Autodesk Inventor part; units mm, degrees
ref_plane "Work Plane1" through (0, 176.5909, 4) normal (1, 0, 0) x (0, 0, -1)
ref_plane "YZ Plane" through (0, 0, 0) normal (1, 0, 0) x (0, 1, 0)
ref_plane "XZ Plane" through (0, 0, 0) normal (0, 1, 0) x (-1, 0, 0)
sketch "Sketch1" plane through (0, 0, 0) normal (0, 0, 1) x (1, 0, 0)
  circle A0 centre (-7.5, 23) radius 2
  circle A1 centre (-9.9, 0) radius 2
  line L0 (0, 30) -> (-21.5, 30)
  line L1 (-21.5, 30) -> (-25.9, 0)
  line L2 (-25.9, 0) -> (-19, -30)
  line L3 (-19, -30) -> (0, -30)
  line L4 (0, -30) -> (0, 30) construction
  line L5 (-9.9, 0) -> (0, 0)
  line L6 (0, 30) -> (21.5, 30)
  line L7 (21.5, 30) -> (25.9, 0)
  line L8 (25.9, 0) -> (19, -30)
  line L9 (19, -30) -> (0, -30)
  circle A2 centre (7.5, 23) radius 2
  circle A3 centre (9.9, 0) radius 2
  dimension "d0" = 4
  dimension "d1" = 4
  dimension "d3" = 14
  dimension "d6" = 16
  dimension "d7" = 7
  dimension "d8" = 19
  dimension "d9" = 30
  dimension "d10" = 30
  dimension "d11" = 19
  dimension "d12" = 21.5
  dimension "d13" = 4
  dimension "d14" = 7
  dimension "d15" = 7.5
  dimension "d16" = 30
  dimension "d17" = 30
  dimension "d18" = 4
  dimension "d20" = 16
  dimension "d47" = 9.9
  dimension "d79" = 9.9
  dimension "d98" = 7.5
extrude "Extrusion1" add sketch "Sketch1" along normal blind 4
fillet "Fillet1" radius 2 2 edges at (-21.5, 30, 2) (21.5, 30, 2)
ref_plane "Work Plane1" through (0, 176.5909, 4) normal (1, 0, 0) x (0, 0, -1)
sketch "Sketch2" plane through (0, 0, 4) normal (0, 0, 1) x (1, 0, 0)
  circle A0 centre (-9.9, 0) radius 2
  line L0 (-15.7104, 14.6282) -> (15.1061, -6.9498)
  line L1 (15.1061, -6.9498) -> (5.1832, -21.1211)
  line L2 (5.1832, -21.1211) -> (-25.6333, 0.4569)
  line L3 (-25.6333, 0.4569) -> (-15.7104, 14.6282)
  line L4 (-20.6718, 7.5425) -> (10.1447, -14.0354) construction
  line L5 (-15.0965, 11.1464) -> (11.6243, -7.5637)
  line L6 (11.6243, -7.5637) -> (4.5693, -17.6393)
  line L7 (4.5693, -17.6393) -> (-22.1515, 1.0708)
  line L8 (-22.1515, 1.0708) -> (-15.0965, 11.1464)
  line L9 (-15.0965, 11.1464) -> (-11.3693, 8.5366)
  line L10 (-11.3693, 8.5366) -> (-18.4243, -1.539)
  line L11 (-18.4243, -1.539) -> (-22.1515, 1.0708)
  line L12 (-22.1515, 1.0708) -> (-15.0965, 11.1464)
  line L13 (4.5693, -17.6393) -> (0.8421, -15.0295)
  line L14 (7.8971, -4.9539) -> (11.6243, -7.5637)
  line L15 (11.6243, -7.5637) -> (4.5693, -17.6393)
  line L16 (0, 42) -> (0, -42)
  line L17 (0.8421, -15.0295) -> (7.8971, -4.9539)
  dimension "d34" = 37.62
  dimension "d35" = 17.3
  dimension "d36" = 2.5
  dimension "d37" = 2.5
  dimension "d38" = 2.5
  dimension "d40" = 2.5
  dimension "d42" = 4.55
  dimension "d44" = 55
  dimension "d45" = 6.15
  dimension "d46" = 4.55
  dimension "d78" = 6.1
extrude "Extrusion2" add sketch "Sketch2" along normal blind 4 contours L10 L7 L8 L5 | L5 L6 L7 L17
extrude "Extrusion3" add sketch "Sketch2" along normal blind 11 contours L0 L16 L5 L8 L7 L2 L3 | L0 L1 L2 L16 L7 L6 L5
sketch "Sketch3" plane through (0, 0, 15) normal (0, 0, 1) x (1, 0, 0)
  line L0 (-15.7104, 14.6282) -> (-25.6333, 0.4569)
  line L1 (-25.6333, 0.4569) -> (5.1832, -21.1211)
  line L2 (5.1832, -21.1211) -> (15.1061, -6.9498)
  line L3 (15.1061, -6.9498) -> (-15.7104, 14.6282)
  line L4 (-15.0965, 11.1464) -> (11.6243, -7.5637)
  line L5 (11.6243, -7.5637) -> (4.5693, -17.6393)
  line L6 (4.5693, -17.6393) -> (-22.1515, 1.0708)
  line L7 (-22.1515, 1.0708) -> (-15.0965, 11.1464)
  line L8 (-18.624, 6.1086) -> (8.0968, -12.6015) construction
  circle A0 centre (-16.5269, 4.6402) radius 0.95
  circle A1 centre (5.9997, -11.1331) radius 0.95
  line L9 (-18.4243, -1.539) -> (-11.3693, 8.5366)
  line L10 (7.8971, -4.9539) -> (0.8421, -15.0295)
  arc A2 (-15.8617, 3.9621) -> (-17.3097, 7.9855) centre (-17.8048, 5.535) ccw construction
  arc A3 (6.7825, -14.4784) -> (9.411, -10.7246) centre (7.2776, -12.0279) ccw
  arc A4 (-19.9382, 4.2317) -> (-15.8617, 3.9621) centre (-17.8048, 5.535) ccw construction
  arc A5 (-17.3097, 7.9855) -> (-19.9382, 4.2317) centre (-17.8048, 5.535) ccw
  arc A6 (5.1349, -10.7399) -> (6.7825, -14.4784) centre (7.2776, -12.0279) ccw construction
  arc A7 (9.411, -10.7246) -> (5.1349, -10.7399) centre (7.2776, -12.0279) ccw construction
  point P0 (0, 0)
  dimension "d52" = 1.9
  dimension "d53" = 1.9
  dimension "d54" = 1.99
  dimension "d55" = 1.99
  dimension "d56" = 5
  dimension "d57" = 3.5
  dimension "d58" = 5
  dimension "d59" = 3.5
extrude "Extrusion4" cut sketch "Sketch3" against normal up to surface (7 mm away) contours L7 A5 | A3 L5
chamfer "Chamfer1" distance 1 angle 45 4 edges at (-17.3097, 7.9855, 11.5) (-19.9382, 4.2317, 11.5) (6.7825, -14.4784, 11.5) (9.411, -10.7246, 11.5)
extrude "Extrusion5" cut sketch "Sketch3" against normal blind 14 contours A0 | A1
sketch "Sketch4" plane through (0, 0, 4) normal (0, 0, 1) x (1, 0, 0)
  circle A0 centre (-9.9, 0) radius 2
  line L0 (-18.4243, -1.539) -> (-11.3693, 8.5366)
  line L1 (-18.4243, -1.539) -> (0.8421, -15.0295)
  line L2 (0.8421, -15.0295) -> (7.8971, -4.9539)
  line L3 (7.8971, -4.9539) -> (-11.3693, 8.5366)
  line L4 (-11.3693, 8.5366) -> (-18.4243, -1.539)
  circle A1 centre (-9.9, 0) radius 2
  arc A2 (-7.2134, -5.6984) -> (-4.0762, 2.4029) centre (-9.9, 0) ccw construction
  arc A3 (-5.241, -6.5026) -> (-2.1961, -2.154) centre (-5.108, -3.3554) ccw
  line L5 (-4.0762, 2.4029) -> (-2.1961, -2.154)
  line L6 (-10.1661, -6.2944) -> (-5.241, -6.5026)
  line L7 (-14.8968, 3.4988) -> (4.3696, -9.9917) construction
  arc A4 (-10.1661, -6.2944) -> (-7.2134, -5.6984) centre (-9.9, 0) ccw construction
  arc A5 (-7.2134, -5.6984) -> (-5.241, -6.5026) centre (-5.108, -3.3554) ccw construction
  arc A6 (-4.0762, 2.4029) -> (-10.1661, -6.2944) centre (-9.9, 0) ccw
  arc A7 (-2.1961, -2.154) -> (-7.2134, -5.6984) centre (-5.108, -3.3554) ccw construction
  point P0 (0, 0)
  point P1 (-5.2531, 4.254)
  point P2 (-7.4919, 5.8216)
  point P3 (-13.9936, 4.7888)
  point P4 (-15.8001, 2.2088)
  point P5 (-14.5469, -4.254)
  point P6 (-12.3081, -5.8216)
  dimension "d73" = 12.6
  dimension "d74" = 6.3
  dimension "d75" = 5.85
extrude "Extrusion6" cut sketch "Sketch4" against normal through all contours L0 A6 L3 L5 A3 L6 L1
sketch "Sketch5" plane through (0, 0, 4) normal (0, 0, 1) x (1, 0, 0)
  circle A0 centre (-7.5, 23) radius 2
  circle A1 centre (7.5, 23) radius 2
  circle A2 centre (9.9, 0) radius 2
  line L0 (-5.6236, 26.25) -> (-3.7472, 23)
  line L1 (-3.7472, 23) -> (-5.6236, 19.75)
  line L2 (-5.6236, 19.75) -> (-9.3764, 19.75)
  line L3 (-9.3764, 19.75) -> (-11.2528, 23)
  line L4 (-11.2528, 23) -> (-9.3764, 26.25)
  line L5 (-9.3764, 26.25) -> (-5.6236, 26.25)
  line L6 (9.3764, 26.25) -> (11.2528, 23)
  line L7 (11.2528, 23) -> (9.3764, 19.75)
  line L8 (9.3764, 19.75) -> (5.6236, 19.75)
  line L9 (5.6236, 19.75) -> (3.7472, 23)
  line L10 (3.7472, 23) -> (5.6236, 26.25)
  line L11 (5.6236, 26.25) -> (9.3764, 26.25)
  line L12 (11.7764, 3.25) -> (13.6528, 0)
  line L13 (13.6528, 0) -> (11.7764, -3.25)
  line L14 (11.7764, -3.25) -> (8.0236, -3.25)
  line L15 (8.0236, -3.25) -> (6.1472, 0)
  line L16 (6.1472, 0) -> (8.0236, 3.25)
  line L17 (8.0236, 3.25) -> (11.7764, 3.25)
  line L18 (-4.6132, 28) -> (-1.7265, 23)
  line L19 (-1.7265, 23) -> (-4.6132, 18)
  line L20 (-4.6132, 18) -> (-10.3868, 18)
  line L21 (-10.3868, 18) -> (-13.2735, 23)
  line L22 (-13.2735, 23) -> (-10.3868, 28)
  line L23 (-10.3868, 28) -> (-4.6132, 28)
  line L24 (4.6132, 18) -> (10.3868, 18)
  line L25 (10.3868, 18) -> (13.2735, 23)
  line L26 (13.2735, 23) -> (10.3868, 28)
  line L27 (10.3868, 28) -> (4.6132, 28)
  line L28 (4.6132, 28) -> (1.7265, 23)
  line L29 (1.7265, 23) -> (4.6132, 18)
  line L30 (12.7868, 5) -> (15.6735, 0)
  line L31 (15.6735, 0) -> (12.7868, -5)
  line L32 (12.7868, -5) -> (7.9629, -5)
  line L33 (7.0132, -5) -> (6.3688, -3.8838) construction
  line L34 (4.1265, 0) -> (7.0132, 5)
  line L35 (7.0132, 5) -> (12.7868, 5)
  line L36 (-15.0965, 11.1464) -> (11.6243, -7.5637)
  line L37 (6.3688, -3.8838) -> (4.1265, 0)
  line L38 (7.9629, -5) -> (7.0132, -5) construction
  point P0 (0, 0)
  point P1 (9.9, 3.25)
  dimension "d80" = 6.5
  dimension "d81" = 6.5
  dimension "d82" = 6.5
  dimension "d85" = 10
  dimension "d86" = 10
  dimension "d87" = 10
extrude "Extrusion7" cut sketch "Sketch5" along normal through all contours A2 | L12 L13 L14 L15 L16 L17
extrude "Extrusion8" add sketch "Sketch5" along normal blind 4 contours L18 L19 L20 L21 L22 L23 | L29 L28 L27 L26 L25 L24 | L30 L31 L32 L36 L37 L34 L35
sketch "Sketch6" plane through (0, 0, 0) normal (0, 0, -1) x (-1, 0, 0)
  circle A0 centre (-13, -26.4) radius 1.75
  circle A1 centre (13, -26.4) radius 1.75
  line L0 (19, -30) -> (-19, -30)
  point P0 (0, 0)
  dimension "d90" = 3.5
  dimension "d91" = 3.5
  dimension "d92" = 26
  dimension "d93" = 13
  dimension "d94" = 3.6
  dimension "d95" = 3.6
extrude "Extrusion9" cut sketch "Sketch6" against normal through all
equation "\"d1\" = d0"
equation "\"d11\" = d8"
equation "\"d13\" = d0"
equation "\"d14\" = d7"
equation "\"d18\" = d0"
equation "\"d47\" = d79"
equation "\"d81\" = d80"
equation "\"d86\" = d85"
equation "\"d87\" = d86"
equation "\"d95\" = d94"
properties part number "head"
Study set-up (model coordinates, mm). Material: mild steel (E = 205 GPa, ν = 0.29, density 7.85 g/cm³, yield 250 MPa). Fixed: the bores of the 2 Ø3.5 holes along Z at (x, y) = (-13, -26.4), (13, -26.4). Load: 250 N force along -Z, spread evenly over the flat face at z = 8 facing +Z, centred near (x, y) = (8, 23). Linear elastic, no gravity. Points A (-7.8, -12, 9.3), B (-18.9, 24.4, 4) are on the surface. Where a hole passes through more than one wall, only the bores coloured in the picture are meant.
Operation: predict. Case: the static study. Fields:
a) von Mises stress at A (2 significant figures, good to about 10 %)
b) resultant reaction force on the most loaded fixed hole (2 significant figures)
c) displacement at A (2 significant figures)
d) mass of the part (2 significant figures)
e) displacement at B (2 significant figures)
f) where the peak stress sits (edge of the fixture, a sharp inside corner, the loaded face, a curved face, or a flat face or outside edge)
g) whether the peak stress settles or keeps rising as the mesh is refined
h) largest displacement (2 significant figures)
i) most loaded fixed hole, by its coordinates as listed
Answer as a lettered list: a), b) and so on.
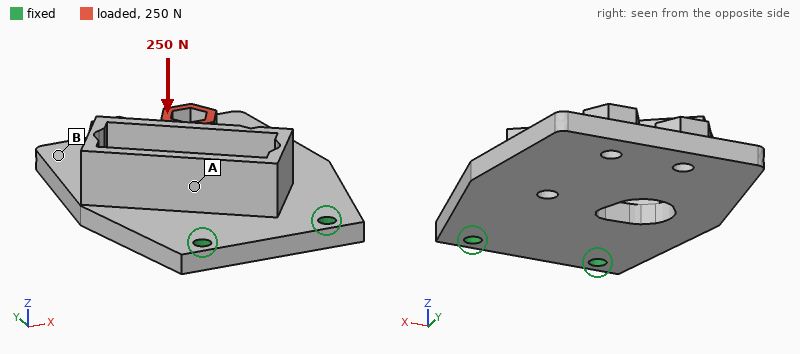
a) 25 MPa
b) 180 N
c) 0.036 mm
d) 110 g
e) 0.17 mm
f) edge of the fixture
g) keeps rising
h) 0.23 mm
i) (13, -26.4)
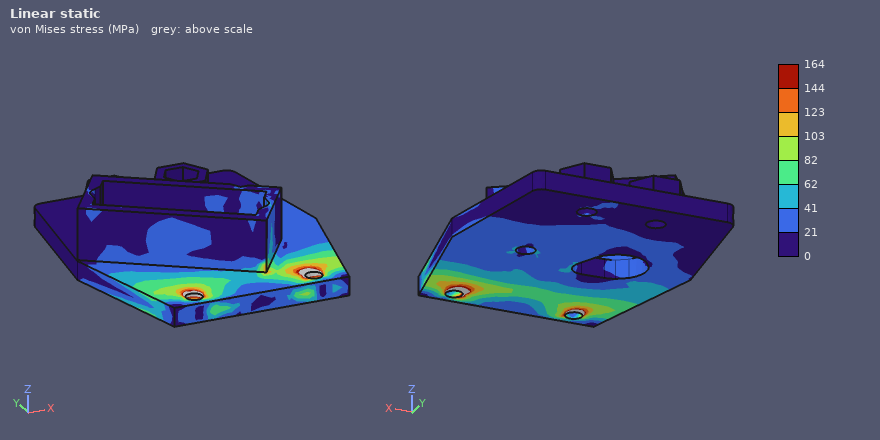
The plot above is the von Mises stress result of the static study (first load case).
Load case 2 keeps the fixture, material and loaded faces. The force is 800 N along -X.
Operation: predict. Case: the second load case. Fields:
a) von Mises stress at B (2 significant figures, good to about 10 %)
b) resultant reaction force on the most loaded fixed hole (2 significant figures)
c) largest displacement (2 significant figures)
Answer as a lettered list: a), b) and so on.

a) 11 MPa
b) 1.5 kN
c) 41 µm
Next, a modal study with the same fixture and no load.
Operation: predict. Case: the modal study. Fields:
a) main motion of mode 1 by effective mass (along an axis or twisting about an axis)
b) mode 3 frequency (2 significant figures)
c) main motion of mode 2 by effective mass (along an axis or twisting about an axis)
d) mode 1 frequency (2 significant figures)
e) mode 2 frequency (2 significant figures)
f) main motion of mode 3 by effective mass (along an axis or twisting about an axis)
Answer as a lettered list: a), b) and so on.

a) along Z
b) 5800 Hz
c) twisting about Y
d) 980 Hz
e) 3500 Hz
f) along X
